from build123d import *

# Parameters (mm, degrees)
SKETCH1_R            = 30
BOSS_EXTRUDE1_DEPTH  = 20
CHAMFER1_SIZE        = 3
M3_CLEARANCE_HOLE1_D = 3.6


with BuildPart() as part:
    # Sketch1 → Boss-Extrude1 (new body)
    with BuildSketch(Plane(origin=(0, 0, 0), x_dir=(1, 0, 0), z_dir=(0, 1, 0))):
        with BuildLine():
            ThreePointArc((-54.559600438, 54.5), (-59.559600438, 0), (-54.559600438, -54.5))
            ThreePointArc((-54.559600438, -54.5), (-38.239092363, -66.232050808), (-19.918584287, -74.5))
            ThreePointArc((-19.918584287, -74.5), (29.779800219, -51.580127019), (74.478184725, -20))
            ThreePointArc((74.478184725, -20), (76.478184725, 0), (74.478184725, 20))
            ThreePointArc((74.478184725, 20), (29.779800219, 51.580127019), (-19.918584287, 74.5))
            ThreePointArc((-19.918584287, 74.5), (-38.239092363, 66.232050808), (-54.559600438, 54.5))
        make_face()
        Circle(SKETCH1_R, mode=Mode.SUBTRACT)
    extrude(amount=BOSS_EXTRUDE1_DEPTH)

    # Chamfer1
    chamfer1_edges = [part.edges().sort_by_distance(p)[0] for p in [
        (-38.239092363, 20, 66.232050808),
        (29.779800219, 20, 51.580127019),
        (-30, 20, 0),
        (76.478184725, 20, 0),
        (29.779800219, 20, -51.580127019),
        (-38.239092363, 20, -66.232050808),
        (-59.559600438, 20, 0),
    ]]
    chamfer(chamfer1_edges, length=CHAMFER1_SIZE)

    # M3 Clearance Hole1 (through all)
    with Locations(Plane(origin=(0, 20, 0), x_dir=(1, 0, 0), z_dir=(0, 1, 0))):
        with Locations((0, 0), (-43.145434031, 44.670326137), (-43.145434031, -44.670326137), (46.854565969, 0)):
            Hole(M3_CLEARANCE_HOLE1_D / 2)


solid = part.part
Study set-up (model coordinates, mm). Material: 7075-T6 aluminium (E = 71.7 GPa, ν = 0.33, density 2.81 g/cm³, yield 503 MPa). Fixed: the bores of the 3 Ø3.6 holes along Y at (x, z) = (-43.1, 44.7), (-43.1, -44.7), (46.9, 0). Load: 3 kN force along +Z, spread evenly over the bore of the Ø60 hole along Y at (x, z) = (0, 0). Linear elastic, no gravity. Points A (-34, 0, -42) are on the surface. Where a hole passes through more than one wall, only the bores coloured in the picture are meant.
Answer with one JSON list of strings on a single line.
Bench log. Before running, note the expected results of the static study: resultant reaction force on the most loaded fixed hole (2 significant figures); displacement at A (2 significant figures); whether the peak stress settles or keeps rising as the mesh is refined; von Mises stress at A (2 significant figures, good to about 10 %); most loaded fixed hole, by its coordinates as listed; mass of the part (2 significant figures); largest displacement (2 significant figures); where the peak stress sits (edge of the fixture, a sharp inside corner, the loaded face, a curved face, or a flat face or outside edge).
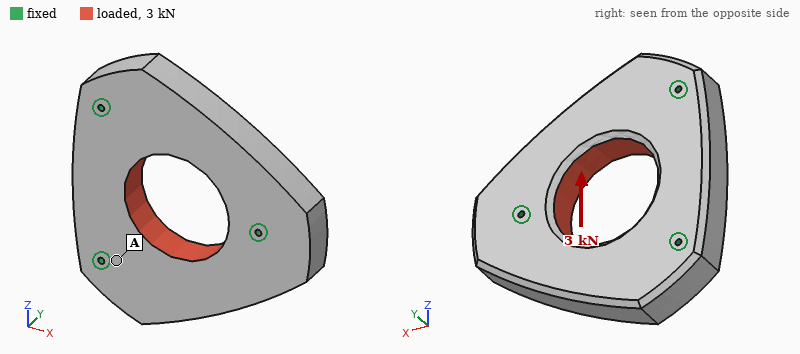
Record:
["1.5 kN", "0.52 µm", "keeps rising", "1.1 MPa", "(46.9, 0)", "650 g", "2.0 µm", "edge of the fixture"]
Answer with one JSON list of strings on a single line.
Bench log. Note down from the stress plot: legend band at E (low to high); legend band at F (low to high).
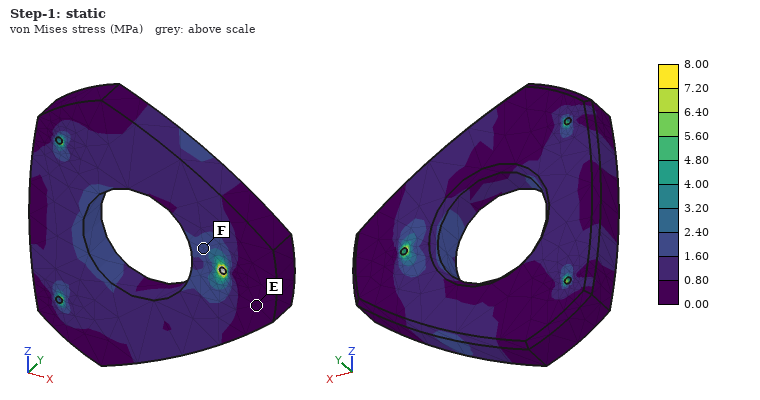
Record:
["0.00 to 0.80 MPa", "1.60 to 2.40 MPa"]
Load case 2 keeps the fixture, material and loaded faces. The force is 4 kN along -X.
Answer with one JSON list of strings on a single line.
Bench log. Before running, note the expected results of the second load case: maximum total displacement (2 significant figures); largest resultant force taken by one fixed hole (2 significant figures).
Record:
["3.0 µm", "1.4 kN"]
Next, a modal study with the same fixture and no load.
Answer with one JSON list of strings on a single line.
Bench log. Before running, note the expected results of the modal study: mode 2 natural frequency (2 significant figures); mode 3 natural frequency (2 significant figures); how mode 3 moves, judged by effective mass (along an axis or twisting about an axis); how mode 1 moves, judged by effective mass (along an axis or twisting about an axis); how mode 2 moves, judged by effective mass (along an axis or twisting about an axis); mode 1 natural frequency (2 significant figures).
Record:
["5200 Hz", "8000 Hz", "along Y", "twisting about X", "along Y", "4500 Hz"]
